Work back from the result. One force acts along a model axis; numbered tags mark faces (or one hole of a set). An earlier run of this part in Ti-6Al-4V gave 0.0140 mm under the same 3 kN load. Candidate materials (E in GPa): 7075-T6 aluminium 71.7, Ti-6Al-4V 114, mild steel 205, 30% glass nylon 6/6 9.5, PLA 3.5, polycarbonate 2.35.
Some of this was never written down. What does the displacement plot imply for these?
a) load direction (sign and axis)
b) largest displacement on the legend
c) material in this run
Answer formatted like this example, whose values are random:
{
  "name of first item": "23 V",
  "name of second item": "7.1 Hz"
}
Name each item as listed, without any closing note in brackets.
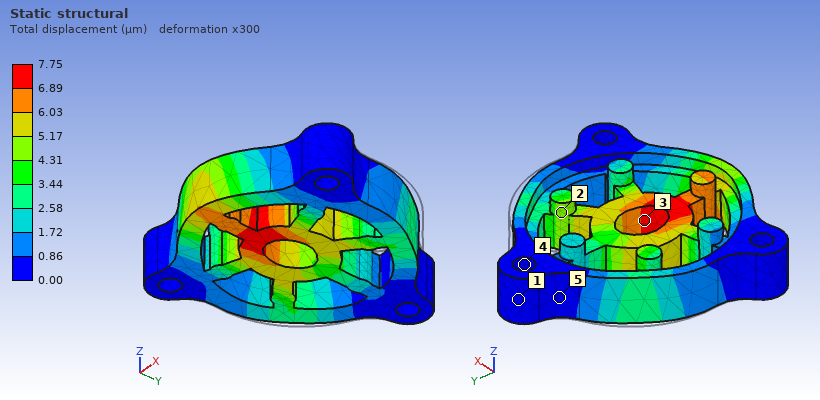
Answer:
{
  "load direction": "-Y",
  "largest displacement on the legend": "7.75 µm",
  "material in this run": "mild steel"
}
